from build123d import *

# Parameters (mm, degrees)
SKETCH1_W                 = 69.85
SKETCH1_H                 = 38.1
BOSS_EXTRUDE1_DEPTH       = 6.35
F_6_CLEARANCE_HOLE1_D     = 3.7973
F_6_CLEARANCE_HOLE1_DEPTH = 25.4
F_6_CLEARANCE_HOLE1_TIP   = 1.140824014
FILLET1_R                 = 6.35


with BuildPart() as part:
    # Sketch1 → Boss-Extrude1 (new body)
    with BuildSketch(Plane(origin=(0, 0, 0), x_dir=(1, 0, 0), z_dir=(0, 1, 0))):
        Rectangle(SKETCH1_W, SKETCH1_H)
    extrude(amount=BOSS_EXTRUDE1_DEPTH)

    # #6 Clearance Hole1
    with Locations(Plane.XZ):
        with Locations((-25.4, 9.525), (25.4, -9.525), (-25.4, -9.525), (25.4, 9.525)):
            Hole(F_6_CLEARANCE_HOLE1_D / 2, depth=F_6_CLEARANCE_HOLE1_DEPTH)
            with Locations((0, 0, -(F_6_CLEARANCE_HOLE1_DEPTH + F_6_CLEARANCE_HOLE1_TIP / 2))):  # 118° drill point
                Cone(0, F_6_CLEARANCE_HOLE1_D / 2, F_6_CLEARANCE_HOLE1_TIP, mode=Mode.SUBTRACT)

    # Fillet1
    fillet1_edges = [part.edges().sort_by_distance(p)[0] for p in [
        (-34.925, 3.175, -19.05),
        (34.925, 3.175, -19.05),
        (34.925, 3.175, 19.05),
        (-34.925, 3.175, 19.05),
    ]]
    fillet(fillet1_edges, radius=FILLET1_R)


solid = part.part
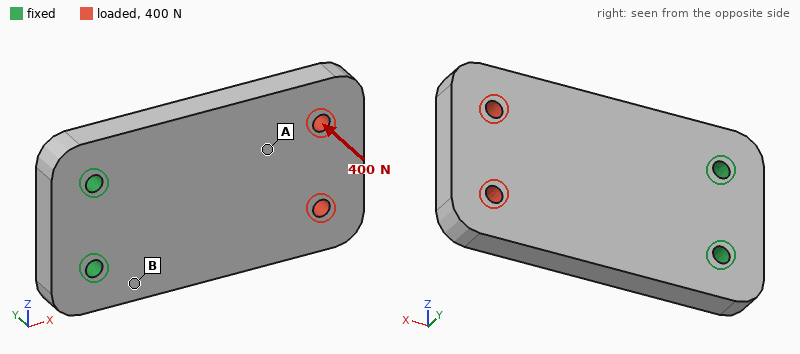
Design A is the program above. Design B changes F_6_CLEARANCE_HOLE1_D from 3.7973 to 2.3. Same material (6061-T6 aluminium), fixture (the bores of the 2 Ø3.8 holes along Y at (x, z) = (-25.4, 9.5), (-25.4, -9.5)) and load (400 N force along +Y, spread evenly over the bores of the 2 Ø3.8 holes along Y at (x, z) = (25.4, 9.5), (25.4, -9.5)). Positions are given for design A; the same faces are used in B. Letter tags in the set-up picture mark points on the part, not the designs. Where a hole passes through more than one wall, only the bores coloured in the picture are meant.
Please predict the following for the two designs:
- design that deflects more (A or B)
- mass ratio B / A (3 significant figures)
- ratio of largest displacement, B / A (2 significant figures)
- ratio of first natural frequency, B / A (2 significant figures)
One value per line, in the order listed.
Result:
B
1.01
1.1
0.93
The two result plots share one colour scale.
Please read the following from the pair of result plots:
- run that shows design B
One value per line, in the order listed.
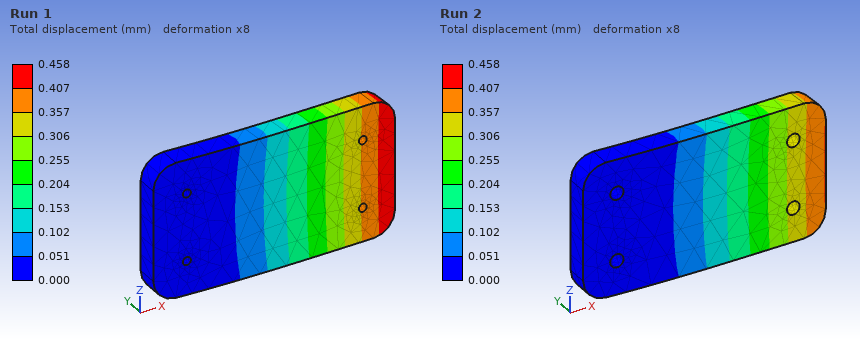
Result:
Run 1
